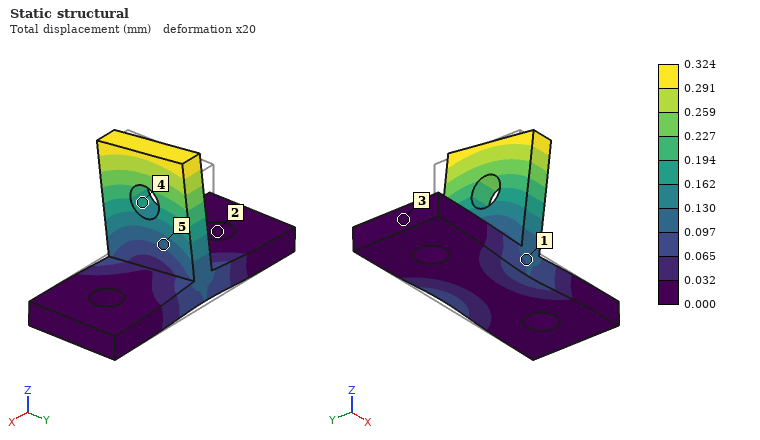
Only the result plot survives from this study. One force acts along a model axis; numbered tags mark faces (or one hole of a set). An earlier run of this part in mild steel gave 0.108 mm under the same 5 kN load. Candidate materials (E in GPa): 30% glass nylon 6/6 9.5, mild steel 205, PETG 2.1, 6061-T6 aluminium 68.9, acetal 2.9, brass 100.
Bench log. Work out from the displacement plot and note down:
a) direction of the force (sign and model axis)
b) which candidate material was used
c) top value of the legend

-Y
6061-T6 aluminium
0.324 mm
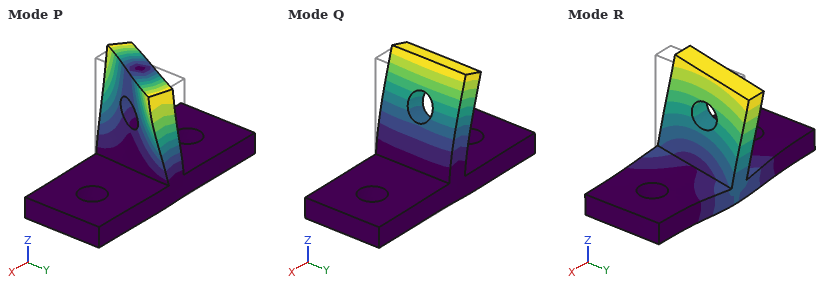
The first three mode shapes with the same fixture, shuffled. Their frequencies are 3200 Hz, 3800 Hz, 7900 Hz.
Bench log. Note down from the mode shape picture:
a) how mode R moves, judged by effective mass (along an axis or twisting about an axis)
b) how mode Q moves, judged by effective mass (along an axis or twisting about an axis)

along Y
along X
